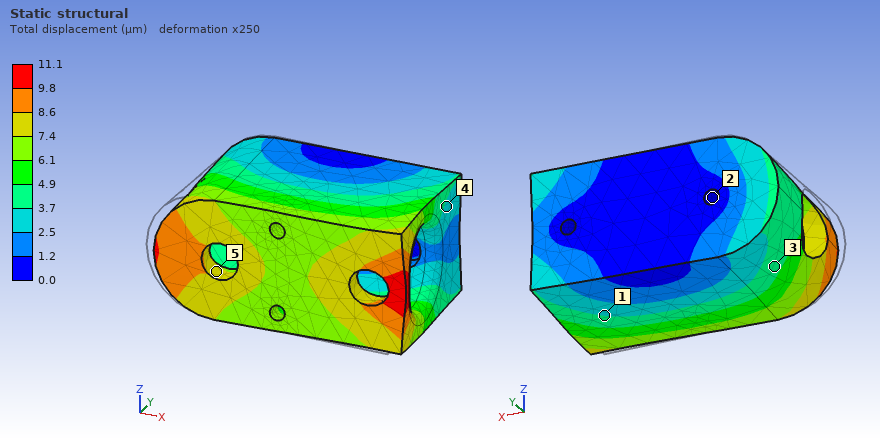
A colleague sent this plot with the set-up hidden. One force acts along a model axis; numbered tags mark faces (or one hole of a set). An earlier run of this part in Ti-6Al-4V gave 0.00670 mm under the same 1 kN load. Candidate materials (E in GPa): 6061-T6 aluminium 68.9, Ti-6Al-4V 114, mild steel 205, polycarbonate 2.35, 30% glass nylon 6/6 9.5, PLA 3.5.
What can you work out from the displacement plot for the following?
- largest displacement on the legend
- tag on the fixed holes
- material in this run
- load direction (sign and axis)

11.1 µm
2
6061-T6 aluminium
+X
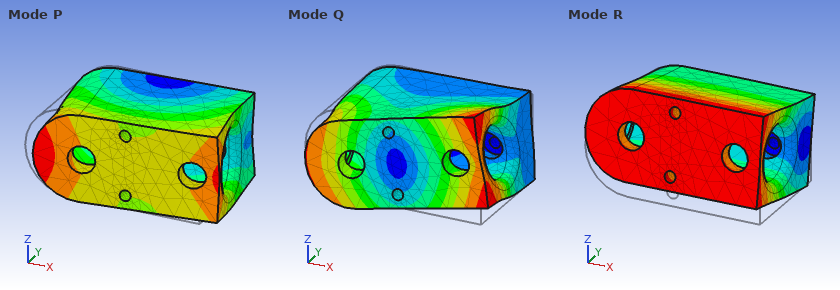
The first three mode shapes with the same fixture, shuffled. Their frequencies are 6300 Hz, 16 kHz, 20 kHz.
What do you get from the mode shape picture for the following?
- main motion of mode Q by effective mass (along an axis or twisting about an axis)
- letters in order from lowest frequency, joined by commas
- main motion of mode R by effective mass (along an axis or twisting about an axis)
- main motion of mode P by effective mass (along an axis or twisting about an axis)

twisting about Y
R, P, Q
along Z
along X
